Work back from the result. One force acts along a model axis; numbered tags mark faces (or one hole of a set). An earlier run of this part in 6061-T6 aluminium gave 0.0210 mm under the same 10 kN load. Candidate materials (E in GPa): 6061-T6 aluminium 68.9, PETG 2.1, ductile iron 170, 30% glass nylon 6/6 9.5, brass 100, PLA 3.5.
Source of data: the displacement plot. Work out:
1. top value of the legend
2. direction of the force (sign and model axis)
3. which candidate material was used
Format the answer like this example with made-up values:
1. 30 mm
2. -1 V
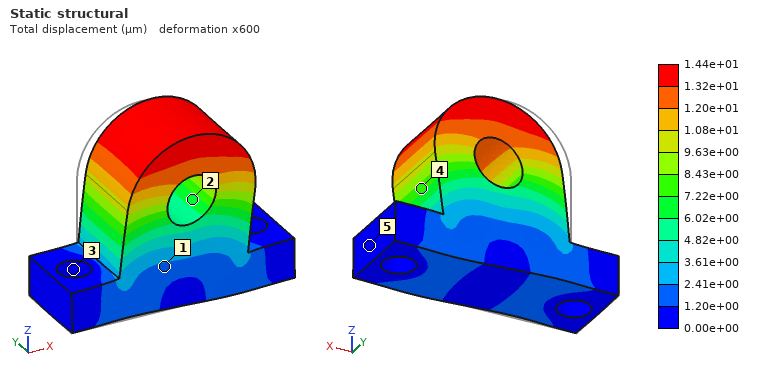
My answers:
1. 1.44e+01 µm
2. +X
3. brass
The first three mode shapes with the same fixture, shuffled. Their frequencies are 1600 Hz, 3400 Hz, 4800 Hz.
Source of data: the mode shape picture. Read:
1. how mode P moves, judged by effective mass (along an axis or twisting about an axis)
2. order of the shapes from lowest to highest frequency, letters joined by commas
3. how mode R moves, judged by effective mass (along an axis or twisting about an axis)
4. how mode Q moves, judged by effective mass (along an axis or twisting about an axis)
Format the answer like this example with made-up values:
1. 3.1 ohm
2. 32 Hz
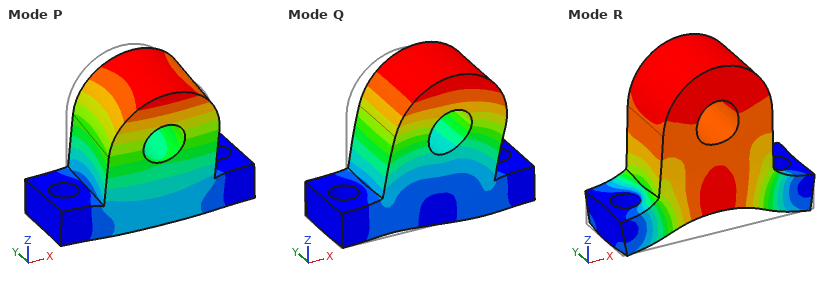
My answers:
1. along Y
2. P, Q, R
3. along Z
4. along X
